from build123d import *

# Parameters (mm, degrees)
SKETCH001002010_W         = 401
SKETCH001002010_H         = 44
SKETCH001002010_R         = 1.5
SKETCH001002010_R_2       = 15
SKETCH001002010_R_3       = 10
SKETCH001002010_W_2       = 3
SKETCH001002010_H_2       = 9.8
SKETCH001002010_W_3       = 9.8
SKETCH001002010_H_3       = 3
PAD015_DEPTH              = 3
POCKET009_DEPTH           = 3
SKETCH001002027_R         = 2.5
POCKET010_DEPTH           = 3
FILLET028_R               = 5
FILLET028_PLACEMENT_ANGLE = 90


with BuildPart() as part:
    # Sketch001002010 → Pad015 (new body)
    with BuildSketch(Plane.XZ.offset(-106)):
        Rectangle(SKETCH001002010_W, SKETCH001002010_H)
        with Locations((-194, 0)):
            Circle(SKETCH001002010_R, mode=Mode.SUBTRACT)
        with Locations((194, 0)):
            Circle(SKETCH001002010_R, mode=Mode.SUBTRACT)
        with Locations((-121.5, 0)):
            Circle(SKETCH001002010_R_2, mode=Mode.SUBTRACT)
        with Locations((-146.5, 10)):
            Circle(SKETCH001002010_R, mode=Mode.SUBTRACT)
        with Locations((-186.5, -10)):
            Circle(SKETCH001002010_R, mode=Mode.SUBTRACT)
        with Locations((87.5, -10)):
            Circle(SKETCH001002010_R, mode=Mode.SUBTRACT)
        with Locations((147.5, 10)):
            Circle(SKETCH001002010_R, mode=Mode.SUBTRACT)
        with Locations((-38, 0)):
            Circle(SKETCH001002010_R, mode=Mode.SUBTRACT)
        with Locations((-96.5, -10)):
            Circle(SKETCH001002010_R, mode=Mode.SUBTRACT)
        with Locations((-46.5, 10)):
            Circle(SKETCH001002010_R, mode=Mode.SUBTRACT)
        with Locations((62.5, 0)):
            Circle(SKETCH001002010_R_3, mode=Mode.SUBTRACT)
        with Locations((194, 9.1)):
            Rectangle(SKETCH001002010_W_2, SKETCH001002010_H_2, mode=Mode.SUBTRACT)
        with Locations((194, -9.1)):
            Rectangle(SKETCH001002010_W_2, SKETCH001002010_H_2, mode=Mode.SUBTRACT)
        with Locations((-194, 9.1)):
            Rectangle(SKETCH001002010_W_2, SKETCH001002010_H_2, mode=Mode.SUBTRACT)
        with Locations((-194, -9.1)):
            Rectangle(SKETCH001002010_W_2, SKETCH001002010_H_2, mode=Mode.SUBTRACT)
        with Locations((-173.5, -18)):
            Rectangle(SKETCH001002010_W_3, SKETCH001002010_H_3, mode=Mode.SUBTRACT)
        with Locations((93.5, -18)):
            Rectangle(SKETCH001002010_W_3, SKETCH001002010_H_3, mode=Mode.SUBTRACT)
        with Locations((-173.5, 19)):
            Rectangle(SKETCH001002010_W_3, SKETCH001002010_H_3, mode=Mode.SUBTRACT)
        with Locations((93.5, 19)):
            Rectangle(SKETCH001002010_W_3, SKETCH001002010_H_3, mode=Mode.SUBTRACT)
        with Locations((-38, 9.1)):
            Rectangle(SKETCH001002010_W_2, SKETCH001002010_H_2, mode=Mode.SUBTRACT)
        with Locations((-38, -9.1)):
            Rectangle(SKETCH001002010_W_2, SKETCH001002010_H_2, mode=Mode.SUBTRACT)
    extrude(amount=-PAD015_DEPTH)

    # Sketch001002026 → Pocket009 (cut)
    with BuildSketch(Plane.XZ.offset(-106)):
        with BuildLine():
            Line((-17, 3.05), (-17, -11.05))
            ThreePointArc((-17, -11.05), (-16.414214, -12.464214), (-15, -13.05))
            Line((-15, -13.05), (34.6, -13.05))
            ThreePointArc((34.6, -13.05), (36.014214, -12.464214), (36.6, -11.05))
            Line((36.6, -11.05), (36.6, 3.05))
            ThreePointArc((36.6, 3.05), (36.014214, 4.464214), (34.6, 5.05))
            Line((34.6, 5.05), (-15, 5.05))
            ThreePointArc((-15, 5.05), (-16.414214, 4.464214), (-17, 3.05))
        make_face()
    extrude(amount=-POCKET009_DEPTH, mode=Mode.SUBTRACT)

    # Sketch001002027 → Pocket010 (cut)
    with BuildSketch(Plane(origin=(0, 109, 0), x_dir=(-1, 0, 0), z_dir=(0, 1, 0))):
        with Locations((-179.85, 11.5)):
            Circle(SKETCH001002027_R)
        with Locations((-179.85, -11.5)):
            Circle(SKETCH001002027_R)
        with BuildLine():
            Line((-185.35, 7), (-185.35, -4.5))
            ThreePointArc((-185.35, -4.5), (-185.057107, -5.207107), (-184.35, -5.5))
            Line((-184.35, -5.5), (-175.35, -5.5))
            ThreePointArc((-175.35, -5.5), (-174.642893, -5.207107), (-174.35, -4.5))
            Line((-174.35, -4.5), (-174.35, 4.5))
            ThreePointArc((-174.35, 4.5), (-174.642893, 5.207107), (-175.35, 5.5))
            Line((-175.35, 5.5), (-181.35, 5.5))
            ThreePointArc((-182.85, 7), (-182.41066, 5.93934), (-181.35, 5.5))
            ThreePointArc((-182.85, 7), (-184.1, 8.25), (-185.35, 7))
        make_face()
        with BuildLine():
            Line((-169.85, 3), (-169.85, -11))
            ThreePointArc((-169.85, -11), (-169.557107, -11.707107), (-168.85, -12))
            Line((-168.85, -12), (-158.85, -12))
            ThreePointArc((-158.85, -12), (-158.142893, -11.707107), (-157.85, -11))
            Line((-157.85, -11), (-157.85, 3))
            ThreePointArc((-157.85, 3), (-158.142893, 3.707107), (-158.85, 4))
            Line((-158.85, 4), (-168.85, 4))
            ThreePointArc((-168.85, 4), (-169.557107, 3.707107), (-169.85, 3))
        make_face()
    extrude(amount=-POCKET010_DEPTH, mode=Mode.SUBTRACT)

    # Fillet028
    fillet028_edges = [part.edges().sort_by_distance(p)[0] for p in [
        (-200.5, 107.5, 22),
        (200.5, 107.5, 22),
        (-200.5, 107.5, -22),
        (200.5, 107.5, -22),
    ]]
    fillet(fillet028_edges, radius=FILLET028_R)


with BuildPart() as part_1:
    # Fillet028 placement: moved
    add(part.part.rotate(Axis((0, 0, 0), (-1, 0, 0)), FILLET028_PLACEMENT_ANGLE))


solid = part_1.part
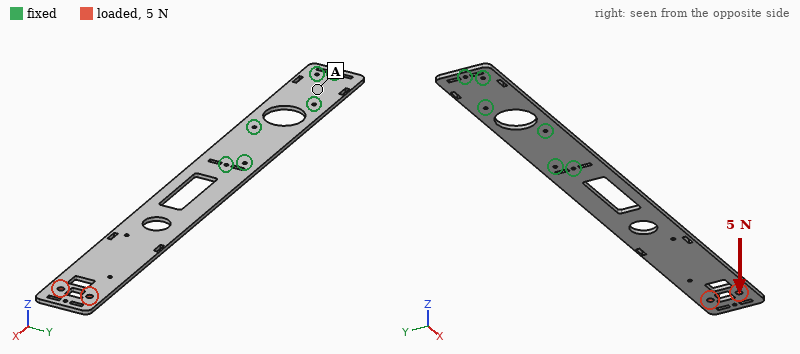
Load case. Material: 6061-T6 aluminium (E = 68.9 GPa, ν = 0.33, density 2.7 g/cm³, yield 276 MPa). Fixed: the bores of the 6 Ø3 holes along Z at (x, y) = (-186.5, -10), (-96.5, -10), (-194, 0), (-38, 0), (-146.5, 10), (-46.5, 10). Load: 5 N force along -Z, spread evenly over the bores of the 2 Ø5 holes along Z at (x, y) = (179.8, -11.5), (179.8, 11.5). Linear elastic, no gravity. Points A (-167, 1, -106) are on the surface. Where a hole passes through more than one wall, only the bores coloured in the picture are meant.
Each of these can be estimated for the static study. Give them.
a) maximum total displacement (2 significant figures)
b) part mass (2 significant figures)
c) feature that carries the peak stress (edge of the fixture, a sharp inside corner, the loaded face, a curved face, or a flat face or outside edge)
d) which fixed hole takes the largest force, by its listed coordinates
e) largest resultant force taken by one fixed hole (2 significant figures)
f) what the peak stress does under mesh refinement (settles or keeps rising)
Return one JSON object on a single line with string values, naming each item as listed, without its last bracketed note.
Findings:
{"maximum total displacement": "4.3 mm", "part mass": "120 g", "feature that carries the peak stress": "edge of the fixture", "which fixed hole takes the largest force, by its listed coordinates": "(-38, 0)", "largest resultant force taken by one fixed hole": "31 N", "what the peak stress does under mesh refinement": "keeps rising"}
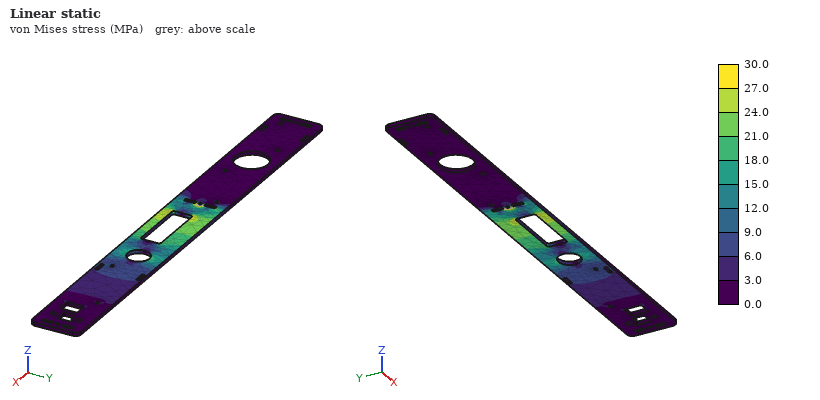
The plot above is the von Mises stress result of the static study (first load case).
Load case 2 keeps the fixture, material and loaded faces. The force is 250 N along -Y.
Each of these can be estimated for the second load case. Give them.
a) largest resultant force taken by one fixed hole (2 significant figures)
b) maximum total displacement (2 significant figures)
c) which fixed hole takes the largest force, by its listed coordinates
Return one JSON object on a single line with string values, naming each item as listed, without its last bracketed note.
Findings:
{"largest resultant force taken by one fixed hole": "1.3 kN", "maximum total displacement": "1.1 mm", "which fixed hole takes the largest force, by its listed coordinates": "(-38, 0)"}
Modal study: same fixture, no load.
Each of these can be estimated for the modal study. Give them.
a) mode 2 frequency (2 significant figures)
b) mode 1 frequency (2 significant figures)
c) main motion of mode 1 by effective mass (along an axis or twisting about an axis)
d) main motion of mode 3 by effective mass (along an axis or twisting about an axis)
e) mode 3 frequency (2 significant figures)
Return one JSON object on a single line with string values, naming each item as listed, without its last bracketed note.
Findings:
{"mode 2 frequency": "260 Hz", "mode 1 frequency": "37 Hz", "main motion of mode 1 by effective mass": "along Z", "main motion of mode 3 by effective mass": "twisting about X", "mode 3 frequency": "370 Hz"}
